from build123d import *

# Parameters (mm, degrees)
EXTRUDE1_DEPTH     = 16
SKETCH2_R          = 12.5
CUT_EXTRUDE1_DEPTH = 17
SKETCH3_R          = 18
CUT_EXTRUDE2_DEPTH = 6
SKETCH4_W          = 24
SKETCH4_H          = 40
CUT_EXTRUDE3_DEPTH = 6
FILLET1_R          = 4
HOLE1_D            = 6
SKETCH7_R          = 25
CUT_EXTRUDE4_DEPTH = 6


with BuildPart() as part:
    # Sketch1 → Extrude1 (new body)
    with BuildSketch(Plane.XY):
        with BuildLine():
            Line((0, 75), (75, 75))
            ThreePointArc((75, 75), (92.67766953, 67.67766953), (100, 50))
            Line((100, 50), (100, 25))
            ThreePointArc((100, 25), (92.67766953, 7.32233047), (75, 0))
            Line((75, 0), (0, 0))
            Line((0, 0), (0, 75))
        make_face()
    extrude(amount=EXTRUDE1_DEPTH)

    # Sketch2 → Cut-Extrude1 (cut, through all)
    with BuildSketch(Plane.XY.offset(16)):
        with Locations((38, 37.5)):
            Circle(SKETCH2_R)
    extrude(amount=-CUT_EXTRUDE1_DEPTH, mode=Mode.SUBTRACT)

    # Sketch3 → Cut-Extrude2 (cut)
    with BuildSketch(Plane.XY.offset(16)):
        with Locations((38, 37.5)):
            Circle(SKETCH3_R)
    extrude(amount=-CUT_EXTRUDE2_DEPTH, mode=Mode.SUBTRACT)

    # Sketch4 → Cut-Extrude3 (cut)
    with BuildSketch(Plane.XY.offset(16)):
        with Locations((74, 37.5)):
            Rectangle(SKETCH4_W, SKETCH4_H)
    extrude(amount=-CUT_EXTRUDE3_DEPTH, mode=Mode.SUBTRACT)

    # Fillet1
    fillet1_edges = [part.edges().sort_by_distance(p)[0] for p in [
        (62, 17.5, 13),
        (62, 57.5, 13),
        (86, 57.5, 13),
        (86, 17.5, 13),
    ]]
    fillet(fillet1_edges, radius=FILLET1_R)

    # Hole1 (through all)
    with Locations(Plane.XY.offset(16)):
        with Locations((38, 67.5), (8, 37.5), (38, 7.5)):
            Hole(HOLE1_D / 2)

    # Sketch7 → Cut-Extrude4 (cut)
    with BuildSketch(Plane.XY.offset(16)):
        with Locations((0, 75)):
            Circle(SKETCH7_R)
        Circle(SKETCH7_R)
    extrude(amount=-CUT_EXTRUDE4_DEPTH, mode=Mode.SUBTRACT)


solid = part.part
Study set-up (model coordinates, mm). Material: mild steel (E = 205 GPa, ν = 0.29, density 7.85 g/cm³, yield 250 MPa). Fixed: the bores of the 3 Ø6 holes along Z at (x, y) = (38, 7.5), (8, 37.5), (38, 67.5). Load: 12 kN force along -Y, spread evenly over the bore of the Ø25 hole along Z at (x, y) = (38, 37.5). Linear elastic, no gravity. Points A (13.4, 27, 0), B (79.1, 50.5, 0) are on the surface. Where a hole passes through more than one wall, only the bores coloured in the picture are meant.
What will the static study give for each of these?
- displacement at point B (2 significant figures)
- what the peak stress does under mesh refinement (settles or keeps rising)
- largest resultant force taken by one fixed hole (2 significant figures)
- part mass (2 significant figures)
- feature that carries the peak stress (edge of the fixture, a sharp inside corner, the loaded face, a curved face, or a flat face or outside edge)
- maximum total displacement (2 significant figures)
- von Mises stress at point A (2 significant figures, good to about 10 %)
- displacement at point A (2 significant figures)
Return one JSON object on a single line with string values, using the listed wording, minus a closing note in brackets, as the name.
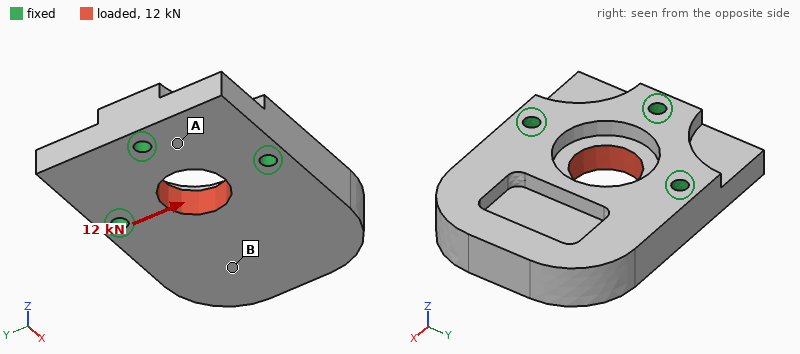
{"displacement at point B": "1.9 µm", "what the peak stress does under mesh refinement": "keeps rising", "largest resultant force taken by one fixed hole": "4.9 kN", "part mass": "720 g", "feature that carries the peak stress": "edge of the fixture", "maximum total displacement": "2.9 µm", "von Mises stress at point A": "6.5 MPa", "displacement at point A": "0.69 µm"}
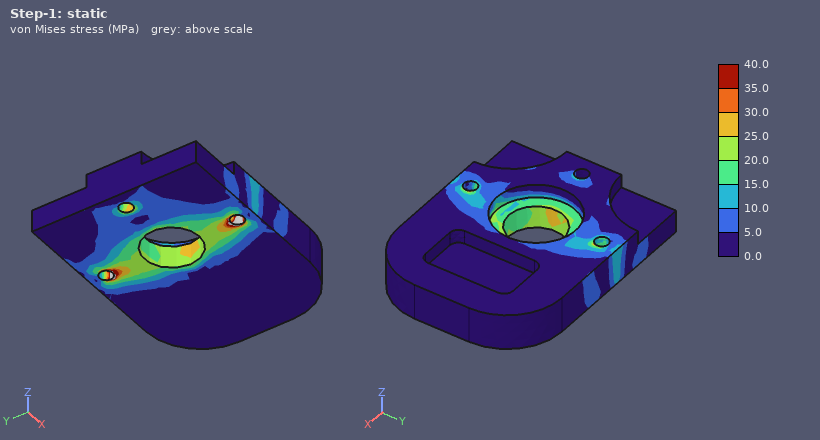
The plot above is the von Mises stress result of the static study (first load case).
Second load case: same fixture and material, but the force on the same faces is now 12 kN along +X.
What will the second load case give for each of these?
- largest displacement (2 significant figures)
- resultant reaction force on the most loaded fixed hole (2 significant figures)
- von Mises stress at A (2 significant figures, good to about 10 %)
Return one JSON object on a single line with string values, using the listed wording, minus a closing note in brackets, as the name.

{"largest displacement": "6.2 µm", "resultant reaction force on the most loaded fixed hole": "4.1 kN", "von Mises stress at A": "9.2 MPa"}
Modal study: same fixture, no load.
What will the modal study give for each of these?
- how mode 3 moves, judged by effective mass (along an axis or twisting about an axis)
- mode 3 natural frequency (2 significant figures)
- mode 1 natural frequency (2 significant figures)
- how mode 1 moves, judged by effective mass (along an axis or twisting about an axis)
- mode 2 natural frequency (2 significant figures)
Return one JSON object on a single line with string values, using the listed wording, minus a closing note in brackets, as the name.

{"how mode 3 moves, judged by effective mass": "along Y", "mode 3 natural frequency": "9100 Hz", "mode 1 natural frequency": "2900 Hz", "how mode 1 moves, judged by effective mass": "along Z", "mode 2 natural frequency": "6300 Hz"}
